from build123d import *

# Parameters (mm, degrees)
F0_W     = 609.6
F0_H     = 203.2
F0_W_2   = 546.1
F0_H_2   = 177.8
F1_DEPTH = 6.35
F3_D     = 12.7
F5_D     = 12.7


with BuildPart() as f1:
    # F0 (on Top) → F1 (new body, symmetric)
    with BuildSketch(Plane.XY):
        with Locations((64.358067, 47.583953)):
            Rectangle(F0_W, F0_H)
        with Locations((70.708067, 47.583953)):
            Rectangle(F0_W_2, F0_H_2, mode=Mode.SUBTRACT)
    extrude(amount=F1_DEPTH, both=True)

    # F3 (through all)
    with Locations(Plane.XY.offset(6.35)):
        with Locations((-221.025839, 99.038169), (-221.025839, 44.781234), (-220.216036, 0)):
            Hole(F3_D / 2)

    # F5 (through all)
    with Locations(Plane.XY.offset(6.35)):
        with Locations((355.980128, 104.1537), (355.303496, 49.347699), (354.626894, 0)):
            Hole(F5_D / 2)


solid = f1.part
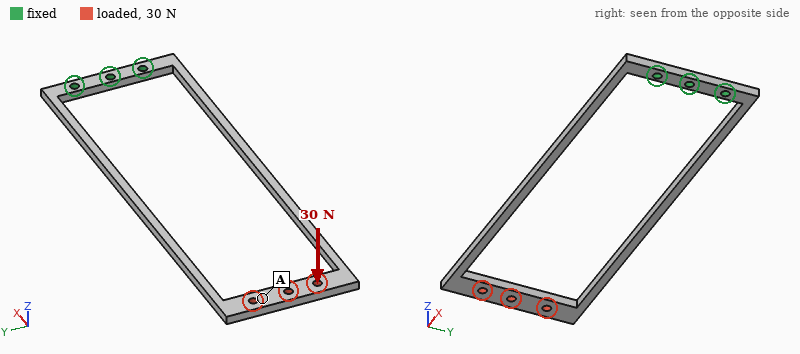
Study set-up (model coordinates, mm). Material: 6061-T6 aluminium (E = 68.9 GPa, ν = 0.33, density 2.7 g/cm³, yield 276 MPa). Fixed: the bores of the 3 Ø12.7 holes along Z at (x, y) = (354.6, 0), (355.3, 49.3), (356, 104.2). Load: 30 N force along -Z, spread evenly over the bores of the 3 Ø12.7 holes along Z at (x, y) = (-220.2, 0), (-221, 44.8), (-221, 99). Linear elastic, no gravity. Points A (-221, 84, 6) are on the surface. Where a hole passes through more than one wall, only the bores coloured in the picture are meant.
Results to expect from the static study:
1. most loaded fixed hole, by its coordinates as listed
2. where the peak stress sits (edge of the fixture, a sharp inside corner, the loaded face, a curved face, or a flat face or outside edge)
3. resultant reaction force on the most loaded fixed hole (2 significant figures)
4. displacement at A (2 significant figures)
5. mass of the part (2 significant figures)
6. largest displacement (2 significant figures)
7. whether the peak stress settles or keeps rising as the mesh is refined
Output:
(356, 104.2)
a sharp inside corner
14 N
6.8 mm
890 g
7.2 mm
keeps rising
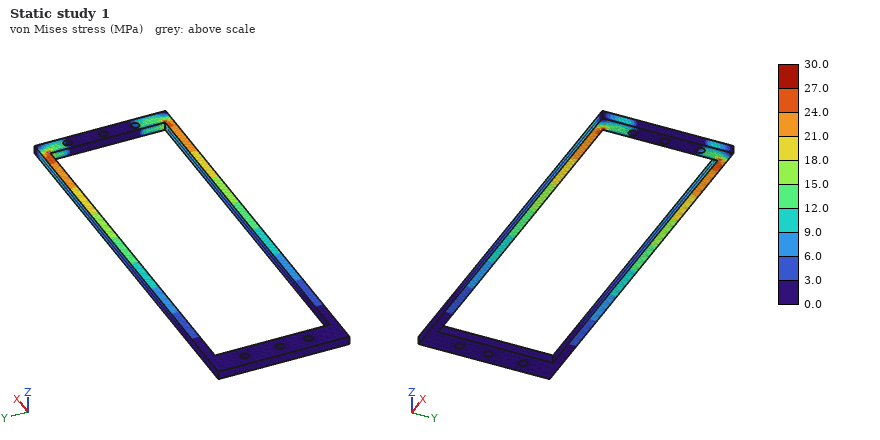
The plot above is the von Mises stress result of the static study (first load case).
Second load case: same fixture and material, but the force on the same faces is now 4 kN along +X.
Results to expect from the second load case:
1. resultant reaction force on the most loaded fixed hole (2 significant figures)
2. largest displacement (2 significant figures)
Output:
2.4 kN
0.40 mm
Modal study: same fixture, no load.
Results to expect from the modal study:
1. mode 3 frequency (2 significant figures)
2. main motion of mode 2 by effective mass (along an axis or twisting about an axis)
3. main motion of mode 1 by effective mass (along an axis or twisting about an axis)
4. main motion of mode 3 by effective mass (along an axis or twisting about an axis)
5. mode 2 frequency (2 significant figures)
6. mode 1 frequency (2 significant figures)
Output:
69 Hz
along Y
along Z
twisting about X
34 Hz
18 Hz
